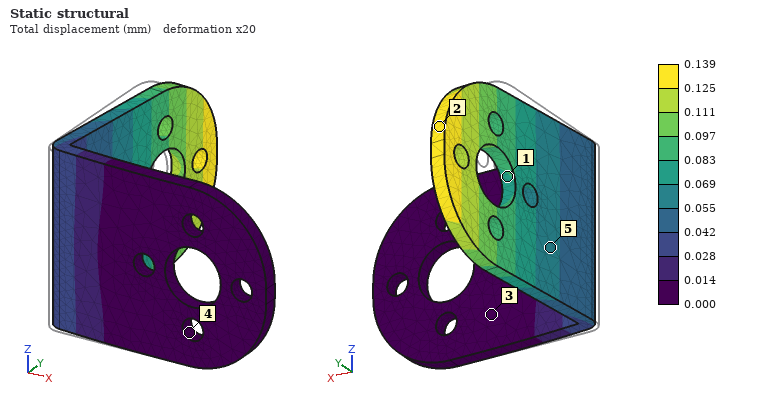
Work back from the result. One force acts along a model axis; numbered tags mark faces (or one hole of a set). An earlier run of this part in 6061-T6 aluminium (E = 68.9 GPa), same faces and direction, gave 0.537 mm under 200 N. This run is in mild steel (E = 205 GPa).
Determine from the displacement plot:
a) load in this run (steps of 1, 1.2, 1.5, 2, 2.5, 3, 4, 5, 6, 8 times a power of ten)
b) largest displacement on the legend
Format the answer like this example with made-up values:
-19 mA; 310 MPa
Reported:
150 N; 0.139 mm
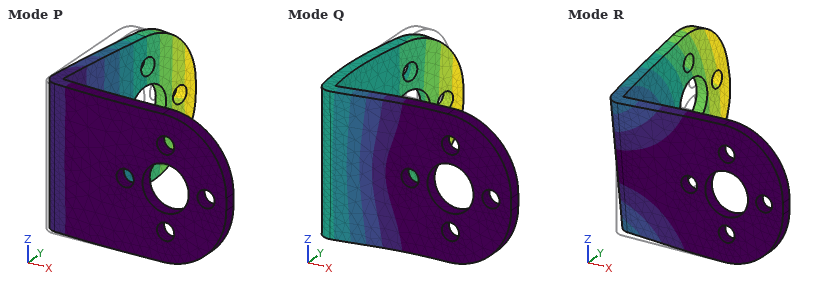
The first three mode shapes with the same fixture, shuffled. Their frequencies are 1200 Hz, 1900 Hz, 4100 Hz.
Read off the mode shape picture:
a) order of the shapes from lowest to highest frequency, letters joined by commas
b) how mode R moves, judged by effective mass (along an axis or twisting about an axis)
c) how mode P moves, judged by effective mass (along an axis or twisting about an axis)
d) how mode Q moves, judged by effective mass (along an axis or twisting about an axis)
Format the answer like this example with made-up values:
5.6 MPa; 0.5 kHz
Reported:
P, R, Q; along Z; along X; along Y
